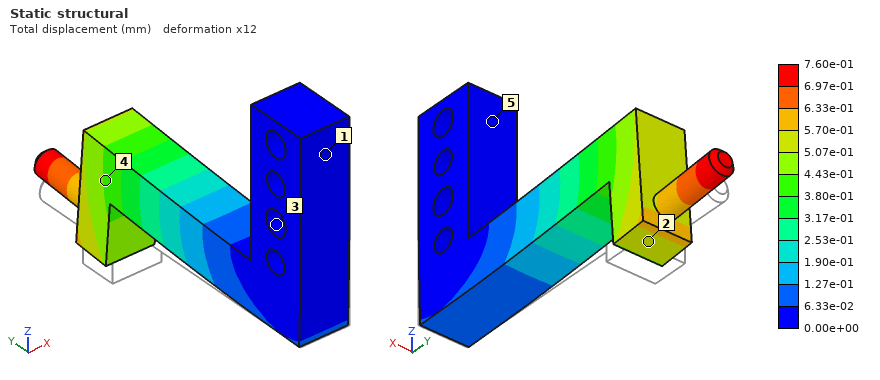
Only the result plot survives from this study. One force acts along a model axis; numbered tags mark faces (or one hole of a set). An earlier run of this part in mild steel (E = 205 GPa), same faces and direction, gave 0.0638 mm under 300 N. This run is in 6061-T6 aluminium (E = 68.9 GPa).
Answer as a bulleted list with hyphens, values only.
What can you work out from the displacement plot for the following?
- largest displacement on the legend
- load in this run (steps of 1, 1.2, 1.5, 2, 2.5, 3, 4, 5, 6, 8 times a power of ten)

- 7.60e-01 mm
- 1.2 kN
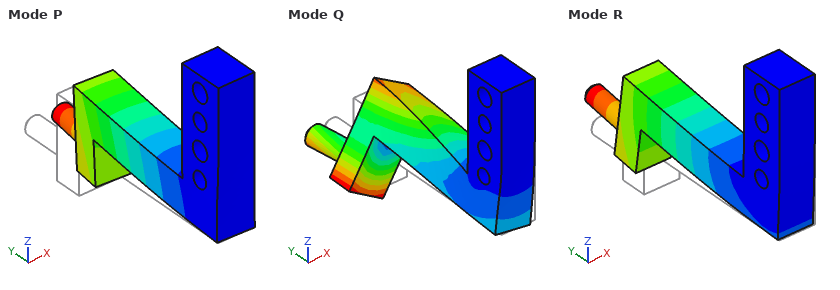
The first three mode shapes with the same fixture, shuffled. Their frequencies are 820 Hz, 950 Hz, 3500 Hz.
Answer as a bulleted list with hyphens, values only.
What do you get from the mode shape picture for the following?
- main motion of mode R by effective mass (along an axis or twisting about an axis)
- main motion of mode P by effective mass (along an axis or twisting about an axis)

- along Z
- along X
